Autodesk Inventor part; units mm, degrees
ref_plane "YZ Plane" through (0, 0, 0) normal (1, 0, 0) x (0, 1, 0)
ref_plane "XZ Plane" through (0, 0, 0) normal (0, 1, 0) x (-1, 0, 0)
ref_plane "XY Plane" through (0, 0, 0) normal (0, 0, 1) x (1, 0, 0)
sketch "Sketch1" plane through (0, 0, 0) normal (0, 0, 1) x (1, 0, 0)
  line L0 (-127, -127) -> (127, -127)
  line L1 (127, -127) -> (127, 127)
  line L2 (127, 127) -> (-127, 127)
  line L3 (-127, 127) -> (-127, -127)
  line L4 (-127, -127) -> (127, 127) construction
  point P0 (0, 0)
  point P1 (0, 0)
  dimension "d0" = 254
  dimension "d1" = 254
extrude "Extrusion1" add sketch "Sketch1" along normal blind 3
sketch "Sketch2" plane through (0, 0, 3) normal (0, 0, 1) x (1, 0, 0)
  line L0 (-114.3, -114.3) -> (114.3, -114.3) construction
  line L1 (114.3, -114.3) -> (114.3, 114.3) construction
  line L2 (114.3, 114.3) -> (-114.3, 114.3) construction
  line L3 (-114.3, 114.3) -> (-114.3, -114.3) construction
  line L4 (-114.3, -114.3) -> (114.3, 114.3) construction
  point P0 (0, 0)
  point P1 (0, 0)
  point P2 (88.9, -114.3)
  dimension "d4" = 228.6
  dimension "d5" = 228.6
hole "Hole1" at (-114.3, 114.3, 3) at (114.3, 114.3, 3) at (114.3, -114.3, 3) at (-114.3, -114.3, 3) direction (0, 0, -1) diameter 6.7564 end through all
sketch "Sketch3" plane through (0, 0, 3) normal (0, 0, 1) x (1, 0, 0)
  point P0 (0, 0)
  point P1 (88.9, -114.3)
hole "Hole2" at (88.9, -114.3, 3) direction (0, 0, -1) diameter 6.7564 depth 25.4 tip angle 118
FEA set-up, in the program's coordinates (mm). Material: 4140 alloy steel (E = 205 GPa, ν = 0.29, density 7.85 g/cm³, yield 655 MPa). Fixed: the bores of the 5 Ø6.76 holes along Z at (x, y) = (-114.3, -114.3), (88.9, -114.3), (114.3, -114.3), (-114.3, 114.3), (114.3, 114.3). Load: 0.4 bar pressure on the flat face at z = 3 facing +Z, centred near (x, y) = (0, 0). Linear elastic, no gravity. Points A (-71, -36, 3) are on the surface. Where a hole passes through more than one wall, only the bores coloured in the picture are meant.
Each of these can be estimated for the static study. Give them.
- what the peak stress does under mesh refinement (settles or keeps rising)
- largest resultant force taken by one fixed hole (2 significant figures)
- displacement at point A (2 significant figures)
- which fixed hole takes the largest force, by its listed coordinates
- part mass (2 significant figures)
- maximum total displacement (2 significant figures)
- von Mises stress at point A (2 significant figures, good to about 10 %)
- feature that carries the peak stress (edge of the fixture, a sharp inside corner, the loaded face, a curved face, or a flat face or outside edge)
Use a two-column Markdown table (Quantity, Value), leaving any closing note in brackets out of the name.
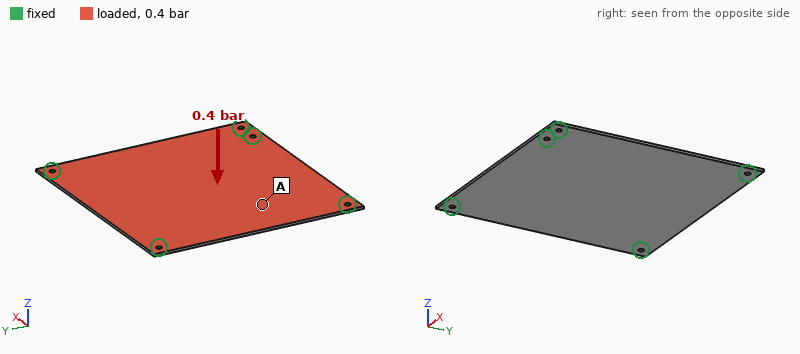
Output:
| Quantity | Value |
|---|---|
| what the peak stress does under mesh refinement | keeps rising |
| largest resultant force taken by one fixed hole | 820 N |
| displacement at point A | 1.2 mm |
| which fixed hole takes the largest force, by its listed coordinates | (88.9, -114.3) |
| part mass | 1.5 kg |
| maximum total displacement | 1.6 mm |
| von Mises stress at point A | 58 MPa |
| feature that carries the peak stress | edge of the fixture |
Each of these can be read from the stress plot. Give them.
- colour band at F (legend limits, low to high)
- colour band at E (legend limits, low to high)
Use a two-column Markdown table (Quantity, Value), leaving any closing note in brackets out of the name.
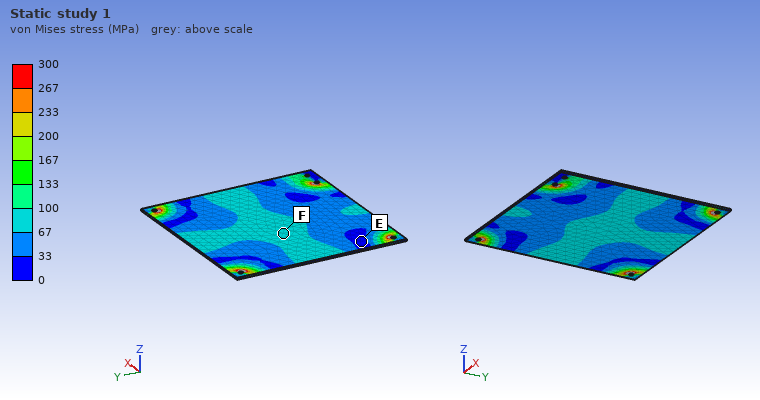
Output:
| Quantity | Value |
|---|---|
| colour band at F | 67 to 100 MPa |
| colour band at E | 0 to 33 MPa |
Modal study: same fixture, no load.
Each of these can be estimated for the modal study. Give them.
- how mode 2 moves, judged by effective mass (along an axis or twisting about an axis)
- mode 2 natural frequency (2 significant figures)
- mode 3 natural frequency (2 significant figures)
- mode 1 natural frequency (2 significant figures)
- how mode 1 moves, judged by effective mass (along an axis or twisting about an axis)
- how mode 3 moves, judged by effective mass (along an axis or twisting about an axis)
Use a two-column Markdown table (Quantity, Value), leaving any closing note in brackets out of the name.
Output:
| Quantity | Value |
|---|---|
| how mode 2 moves, judged by effective mass | twisting about Y |
| mode 2 natural frequency | 330 Hz |
| mode 3 natural frequency | 350 Hz |
| mode 1 natural frequency | 200 Hz |
| how mode 1 moves, judged by effective mass | along Z |
| how mode 3 moves, judged by effective mass | twisting about X |
